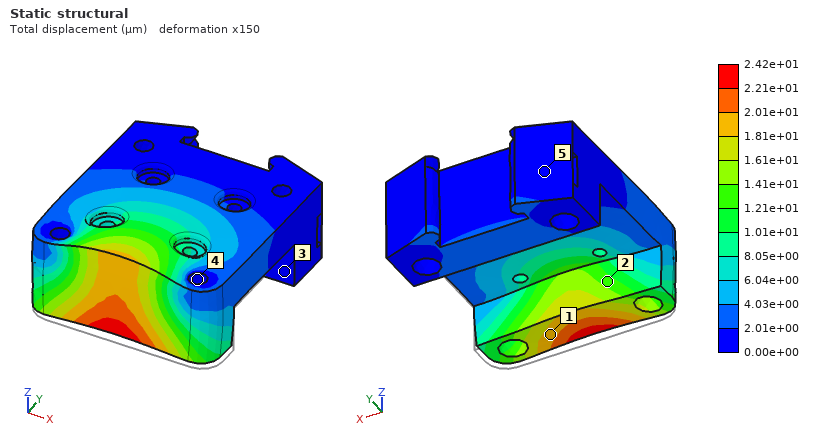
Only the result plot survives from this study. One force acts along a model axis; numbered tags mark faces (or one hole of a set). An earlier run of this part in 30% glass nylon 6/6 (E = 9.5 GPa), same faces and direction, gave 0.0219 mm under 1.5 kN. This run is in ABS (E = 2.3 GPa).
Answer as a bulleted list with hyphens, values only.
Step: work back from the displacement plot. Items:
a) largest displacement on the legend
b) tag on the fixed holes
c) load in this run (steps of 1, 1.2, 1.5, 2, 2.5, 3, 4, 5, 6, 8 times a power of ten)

- 2.42e+01 µm
- 4
- 400 N
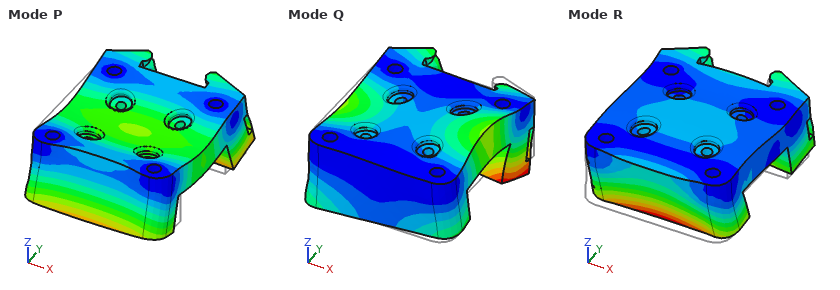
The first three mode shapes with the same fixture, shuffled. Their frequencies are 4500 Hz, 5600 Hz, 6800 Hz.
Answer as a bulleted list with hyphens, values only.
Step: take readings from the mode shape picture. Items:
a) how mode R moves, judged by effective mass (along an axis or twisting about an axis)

- along Y
